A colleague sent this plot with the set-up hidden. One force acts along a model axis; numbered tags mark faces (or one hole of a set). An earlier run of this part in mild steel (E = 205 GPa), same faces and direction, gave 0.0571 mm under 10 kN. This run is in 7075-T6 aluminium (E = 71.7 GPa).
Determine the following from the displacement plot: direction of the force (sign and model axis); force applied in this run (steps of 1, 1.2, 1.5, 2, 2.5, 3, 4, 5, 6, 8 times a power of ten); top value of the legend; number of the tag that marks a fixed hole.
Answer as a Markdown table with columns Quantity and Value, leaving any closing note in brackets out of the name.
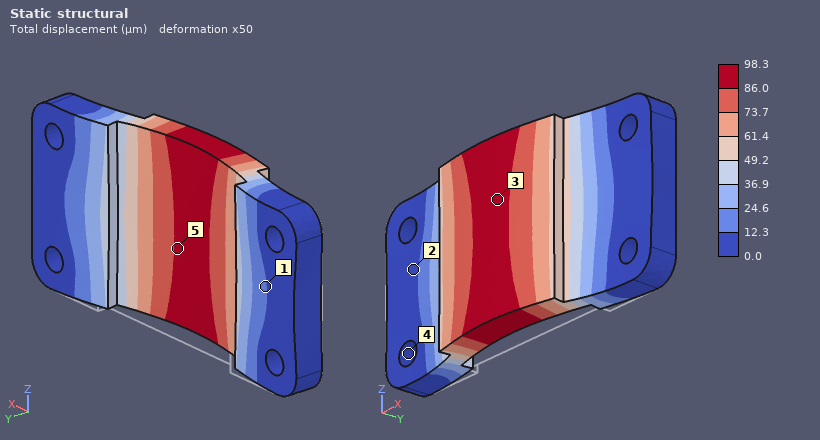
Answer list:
| Quantity | Value |
|---|---|
| direction of the force | -Y |
| force applied in this run | 6 kN |
| top value of the legend | 98.3 µm |
| number of the tag that marks a fixed hole | 4 |
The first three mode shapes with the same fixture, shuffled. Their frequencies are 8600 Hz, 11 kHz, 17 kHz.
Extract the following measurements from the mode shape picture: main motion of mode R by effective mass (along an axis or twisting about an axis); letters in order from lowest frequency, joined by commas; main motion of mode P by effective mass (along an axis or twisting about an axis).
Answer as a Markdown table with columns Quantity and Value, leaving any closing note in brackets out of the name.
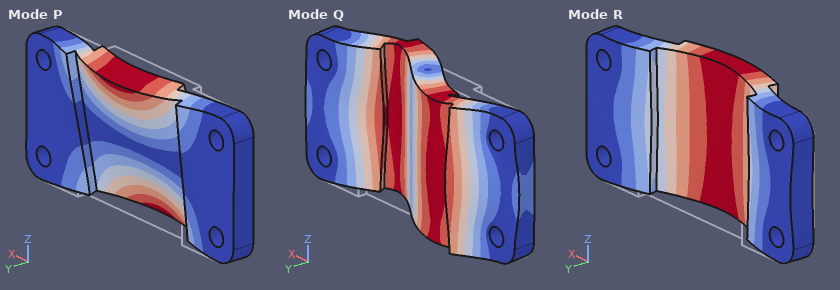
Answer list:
| Quantity | Value |
|---|---|
| main motion of mode R by effective mass | along Y |
| letters in order from lowest frequency, joined by commas | R, P, Q |
| main motion of mode P by effective mass | twisting about X |
